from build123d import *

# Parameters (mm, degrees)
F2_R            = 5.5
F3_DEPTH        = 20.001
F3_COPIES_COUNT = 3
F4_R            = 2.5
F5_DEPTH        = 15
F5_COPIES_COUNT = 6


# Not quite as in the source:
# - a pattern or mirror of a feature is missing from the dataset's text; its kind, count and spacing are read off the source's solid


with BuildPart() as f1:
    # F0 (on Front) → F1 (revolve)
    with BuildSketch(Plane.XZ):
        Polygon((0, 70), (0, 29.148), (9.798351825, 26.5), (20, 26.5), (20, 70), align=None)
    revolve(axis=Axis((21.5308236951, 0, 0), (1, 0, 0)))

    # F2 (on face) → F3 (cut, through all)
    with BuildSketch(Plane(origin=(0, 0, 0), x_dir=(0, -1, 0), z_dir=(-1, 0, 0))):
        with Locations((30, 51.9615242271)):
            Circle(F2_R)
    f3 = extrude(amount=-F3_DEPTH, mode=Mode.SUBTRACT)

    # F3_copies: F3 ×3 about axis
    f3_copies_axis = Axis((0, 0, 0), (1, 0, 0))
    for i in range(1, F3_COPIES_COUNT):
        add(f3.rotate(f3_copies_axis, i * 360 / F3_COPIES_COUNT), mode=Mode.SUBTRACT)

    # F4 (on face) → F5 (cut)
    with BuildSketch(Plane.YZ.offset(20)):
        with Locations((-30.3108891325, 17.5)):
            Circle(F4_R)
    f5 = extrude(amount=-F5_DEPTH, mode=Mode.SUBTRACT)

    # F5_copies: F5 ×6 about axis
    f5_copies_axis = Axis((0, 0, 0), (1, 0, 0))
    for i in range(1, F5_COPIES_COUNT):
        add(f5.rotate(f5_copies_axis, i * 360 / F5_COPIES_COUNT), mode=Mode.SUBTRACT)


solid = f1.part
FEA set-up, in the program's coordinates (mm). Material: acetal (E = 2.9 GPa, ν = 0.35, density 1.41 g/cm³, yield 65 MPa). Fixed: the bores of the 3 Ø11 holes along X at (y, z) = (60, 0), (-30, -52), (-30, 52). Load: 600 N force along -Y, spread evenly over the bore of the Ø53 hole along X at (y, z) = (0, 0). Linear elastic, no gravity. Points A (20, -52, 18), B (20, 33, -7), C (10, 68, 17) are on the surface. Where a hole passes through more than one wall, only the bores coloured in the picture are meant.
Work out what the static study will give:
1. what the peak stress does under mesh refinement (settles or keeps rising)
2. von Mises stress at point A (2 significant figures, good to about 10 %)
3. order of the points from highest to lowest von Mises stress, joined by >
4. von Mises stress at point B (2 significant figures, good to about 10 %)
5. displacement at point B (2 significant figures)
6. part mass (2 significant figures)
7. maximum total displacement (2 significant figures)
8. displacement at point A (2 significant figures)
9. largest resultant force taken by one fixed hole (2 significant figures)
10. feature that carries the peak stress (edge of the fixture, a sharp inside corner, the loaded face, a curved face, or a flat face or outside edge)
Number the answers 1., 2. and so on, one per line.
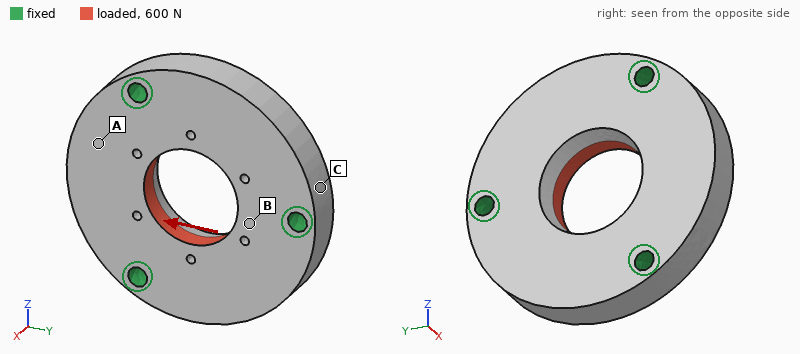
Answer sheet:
1. keeps rising
2. 0.21 MPa
3. B > A > C
4. 0.48 MPa
5. 3.8 µm
6. 360 g
7. 11 µm
8. 7.6 µm
9. 210 N
10. edge of the fixture
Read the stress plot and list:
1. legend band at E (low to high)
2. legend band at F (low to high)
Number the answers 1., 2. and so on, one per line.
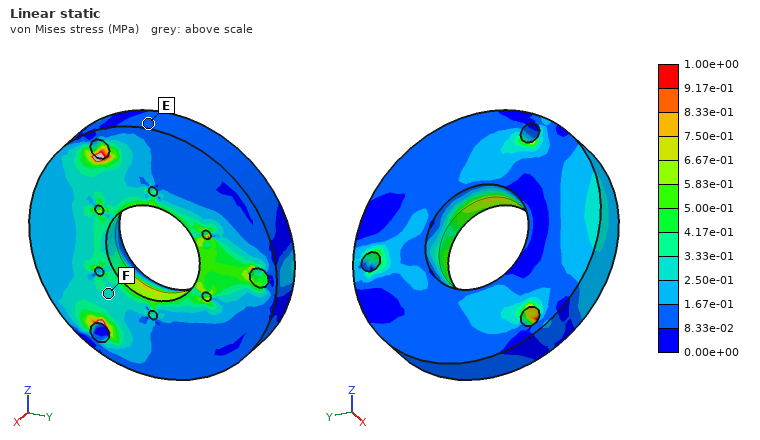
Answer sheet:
1. 8.33e-02 to 1.67e-01 MPa
2. 2.50e-01 to 3.33e-01 MPa
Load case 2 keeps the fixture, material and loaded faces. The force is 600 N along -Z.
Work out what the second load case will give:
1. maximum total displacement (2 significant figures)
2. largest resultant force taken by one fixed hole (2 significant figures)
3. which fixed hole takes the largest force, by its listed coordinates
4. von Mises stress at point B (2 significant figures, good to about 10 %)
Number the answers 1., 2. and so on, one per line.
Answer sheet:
1. 9.5 µm
2. 220 N
3. (60, 0)
4. 0.18 MPa
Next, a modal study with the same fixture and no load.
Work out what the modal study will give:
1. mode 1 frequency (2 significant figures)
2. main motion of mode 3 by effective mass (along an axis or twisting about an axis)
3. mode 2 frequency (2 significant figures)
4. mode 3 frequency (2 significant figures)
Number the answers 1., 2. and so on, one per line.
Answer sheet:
1. 1600 Hz
2. along X
3. 1600 Hz
4. 1800 Hz
